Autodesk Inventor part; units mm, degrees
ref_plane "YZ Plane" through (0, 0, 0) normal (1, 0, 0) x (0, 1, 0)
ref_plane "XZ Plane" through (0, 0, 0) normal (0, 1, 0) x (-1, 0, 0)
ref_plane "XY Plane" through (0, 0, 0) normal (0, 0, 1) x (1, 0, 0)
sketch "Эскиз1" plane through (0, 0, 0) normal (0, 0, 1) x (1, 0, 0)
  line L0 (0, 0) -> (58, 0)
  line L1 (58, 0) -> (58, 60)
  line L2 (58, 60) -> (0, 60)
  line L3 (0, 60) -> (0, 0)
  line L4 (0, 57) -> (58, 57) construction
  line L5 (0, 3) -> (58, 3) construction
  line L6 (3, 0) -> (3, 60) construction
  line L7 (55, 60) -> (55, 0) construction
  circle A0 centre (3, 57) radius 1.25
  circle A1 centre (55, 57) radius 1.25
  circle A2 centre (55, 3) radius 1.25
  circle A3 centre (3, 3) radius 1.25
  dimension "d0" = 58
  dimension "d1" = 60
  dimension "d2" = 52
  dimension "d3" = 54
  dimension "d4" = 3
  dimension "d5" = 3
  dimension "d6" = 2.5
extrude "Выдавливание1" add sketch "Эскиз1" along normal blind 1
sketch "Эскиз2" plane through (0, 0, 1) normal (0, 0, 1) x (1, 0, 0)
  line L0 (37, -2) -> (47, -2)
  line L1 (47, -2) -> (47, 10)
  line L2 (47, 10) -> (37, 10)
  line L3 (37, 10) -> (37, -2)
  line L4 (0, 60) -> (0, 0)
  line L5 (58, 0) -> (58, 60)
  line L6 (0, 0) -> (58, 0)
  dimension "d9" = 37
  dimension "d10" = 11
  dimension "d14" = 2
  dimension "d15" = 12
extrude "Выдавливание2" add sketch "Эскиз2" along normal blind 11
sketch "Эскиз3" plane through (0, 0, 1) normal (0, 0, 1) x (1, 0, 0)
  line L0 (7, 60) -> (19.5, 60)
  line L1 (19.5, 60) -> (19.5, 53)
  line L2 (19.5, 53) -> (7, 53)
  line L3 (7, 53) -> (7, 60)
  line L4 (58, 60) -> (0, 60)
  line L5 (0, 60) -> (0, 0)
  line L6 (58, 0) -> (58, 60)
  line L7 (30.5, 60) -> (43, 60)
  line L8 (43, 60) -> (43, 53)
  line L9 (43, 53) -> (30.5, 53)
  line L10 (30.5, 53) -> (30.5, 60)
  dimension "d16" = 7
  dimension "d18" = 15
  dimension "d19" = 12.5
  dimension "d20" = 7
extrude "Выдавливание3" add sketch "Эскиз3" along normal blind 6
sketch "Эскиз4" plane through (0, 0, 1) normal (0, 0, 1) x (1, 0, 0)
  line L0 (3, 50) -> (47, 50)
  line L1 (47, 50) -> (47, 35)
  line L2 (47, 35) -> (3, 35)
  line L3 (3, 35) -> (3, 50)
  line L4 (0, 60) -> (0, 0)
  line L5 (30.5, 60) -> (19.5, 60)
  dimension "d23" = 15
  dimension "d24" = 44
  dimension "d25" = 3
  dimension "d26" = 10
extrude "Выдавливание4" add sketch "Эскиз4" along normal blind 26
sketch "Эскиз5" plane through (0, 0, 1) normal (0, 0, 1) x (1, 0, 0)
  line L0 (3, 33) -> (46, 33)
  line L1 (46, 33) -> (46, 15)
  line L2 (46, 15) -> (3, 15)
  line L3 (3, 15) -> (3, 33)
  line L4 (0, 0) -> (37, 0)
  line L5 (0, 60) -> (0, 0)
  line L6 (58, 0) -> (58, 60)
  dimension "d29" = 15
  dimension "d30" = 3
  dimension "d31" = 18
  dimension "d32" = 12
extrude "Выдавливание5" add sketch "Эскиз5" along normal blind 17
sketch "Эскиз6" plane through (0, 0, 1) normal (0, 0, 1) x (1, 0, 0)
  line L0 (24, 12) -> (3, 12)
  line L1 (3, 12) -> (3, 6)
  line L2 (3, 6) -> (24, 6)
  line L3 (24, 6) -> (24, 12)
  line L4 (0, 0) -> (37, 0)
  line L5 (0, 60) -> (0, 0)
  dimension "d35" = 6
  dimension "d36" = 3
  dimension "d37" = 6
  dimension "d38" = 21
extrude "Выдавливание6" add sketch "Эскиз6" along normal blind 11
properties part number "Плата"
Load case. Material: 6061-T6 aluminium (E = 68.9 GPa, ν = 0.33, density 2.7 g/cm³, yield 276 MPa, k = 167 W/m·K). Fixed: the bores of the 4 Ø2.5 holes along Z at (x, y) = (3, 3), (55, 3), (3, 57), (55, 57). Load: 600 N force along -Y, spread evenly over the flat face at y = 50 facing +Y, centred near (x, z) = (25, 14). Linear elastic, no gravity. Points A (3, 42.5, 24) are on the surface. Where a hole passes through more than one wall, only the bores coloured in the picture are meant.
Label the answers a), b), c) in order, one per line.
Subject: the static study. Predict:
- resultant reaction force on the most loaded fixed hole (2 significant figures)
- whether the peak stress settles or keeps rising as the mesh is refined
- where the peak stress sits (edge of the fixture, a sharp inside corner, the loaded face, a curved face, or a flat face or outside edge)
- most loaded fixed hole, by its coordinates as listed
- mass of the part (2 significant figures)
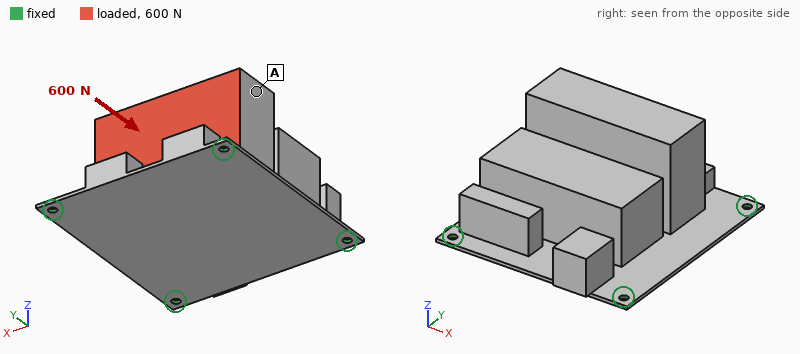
a) 300 N
b) keeps rising
c) edge of the fixture
d) (3, 3)
e) 100 g
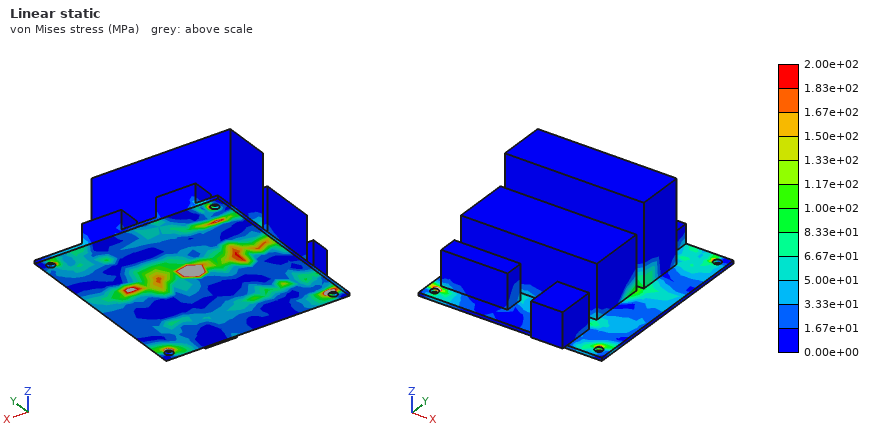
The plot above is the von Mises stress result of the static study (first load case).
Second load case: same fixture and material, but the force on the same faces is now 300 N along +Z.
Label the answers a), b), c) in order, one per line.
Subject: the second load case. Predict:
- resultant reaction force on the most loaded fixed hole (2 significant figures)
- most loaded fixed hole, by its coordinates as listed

a) 190 N
b) (3, 57)
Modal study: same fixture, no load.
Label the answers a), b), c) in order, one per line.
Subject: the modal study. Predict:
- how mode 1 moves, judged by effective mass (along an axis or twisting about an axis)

a) along Z
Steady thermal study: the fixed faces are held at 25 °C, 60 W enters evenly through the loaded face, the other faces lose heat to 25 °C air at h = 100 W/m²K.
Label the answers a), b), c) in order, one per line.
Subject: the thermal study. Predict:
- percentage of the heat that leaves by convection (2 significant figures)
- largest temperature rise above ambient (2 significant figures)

a) 59 %
b) 47 K
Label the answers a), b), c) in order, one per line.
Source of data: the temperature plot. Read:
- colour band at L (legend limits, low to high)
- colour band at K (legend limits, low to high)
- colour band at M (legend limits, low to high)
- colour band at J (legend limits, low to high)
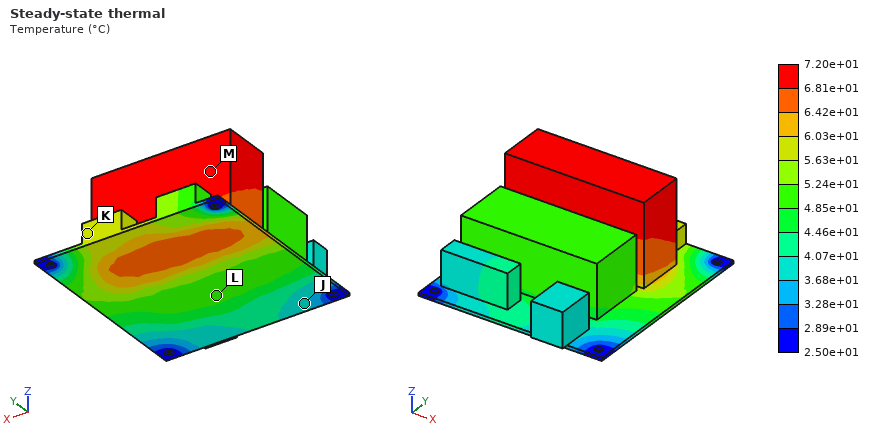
a) 4.85e+01 to 5.24e+01 °C
b) 5.63e+01 to 6.03e+01 °C
c) 6.81e+01 to 7.20e+01 °C
d) 3.68e+01 to 4.07e+01 °C
